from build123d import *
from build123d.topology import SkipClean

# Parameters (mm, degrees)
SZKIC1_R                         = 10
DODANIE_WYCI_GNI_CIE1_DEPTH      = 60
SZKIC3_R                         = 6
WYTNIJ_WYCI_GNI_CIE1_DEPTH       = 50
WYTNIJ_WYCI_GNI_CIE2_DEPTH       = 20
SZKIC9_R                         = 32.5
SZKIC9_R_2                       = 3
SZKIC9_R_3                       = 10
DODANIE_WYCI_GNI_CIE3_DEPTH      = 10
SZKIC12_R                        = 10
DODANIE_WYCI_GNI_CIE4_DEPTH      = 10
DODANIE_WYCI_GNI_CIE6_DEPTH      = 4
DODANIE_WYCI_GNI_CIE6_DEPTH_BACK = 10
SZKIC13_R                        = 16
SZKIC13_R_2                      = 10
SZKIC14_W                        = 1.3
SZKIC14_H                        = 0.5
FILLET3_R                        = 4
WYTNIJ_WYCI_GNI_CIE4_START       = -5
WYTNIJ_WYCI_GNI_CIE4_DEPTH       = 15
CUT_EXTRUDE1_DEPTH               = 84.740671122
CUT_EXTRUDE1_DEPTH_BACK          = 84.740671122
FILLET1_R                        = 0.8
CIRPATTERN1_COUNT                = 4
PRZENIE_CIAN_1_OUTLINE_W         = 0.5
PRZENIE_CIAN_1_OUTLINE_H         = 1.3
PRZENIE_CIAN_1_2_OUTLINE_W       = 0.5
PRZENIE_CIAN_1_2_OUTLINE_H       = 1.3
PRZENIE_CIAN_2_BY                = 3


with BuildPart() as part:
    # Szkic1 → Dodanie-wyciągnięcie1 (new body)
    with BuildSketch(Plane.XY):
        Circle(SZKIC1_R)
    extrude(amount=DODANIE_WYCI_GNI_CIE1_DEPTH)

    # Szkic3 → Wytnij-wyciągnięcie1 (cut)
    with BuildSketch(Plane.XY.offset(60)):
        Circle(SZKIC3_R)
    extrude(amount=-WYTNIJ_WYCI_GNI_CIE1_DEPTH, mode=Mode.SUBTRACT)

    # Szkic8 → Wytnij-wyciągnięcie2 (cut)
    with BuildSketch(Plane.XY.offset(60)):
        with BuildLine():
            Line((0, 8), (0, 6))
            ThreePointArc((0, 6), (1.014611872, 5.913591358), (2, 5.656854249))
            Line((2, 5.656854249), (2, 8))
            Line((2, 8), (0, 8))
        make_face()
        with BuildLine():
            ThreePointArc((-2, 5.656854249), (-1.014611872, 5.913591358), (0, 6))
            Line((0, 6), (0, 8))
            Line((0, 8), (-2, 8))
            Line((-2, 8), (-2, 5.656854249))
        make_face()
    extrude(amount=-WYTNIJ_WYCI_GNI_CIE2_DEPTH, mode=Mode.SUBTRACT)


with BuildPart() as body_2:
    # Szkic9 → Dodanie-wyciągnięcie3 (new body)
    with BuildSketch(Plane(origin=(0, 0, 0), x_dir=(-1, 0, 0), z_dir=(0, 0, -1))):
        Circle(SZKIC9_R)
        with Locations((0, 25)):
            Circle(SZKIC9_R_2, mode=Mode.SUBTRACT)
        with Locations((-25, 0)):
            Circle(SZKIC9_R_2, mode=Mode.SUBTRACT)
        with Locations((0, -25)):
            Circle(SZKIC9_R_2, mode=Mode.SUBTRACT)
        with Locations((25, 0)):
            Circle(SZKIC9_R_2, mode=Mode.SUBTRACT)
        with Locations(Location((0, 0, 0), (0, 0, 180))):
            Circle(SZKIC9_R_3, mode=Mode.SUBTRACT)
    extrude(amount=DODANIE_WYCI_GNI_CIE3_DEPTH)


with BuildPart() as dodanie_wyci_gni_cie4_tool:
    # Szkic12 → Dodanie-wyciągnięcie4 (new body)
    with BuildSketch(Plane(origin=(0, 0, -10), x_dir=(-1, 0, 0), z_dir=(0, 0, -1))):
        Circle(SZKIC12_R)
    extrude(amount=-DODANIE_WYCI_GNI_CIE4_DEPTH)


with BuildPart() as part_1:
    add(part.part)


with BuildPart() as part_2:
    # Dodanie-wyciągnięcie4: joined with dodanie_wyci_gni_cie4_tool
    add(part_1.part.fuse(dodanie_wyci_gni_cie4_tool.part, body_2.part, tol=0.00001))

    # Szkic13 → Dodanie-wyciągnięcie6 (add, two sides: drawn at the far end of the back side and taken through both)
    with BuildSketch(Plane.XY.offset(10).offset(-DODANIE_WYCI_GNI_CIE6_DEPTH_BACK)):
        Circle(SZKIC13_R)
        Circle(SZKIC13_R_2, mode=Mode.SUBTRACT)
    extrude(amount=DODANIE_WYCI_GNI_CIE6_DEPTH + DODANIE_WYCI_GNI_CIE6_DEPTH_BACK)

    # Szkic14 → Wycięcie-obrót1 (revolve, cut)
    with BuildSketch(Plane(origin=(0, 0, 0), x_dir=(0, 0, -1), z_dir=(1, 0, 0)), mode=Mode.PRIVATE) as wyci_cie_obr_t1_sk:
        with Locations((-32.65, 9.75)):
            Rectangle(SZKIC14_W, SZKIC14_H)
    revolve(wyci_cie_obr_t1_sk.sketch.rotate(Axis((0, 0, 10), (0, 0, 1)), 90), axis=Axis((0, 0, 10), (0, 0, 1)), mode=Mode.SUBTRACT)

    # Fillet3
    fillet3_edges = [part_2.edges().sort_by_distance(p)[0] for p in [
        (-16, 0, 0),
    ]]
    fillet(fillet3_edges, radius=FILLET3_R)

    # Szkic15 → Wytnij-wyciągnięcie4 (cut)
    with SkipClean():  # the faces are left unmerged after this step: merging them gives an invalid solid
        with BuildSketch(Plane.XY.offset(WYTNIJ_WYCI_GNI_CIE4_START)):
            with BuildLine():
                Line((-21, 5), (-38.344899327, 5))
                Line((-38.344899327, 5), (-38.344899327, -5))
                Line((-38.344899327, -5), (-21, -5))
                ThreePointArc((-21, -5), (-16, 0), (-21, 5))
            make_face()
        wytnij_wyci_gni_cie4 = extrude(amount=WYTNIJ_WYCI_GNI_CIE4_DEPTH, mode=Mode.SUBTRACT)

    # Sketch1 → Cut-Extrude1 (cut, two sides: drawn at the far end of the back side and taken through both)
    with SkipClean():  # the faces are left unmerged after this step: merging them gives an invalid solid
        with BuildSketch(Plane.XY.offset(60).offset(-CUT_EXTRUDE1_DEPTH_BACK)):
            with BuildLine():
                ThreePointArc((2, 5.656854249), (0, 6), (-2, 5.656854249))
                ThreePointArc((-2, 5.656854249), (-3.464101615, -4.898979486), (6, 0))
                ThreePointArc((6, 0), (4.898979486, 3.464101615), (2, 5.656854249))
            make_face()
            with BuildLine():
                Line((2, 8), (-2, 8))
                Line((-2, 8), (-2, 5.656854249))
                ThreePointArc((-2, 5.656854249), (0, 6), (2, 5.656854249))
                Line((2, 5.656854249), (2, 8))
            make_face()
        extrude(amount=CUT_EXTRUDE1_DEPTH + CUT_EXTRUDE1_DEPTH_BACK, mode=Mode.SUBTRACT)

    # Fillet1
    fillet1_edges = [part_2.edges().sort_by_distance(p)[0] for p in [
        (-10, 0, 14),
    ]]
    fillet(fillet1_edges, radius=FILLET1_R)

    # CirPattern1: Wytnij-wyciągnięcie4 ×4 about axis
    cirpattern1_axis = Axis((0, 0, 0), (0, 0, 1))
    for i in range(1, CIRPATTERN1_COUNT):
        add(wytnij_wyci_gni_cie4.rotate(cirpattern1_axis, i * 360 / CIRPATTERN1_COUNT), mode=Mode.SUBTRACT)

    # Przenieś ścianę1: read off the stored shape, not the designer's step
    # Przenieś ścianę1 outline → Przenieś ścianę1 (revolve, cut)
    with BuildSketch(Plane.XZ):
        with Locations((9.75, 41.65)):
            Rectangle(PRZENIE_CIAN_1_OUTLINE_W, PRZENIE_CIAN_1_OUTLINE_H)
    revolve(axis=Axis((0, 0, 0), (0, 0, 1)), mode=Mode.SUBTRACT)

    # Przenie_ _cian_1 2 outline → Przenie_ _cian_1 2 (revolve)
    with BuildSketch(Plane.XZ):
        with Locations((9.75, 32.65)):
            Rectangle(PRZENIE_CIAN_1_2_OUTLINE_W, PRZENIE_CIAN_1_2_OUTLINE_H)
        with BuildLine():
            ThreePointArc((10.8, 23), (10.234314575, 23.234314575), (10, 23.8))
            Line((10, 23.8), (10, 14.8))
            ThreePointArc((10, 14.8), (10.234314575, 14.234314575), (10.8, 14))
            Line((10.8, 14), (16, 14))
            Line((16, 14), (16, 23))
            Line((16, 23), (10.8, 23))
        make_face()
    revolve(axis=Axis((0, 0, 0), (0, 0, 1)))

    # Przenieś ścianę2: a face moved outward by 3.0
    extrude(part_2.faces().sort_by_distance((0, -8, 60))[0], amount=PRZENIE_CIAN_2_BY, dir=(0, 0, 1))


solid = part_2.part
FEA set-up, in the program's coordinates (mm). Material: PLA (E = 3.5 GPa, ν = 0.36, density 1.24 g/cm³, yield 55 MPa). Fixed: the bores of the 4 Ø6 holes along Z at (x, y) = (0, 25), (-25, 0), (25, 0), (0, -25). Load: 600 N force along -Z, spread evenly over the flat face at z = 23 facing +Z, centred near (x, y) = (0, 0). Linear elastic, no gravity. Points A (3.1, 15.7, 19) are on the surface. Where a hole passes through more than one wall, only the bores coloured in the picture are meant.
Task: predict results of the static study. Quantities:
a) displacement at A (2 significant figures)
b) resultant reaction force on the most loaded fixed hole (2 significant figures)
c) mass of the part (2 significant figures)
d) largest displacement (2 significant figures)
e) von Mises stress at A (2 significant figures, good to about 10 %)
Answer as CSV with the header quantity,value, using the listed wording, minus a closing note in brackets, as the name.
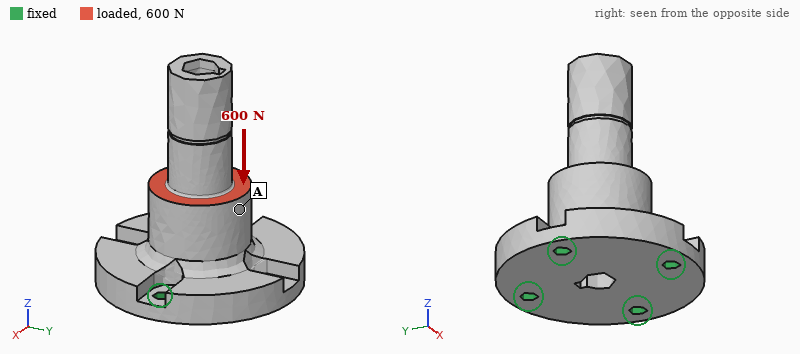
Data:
quantity,value
displacement at A,21 µm
resultant reaction force on the most loaded fixed hole,170 N
mass of the part,65 g
largest displacement,23 µm
von Mises stress at A,1.3 MPa
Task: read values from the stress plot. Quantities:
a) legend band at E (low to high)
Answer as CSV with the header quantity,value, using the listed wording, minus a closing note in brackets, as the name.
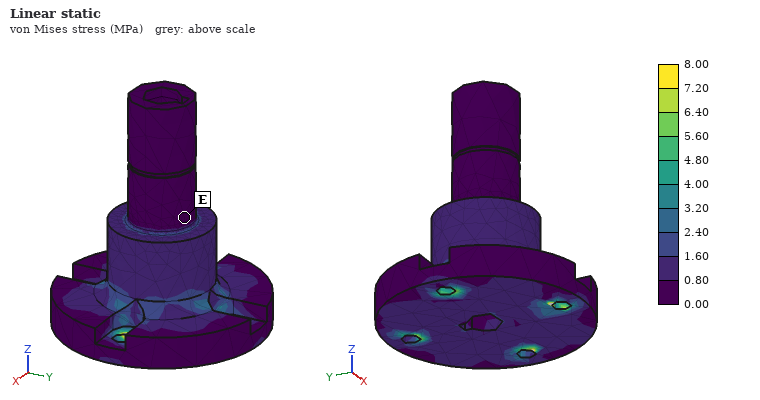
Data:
quantity,value
legend band at E,0.00 to 0.80 MPa
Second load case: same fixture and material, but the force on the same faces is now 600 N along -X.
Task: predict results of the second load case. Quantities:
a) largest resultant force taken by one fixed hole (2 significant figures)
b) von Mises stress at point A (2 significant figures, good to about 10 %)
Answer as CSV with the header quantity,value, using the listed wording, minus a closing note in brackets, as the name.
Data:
quantity,value
largest resultant force taken by one fixed hole,450 N
von Mises stress at point A,1.9 MPa
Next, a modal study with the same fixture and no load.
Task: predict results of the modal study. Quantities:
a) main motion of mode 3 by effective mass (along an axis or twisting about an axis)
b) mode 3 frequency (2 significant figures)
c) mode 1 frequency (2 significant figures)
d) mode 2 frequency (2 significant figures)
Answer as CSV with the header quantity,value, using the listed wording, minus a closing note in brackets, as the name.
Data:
quantity,value
main motion of mode 3 by effective mass,along Z
mode 3 frequency,4300 Hz
mode 1 frequency,1700 Hz
mode 2 frequency,1700 Hz
